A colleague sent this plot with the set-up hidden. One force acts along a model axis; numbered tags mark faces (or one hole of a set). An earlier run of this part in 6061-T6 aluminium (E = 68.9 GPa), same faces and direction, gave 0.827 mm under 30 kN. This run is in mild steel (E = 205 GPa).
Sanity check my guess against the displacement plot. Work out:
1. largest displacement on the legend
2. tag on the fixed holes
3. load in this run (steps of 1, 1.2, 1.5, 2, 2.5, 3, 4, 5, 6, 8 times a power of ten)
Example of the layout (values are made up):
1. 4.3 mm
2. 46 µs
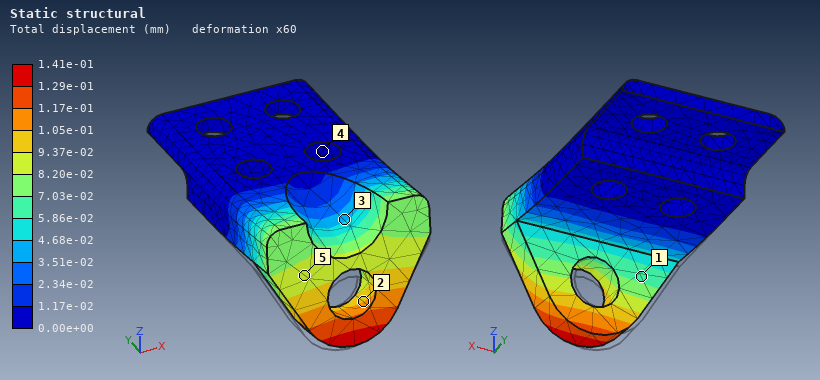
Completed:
1. 1.41e-01 mm
2. 4
3. 15 kN
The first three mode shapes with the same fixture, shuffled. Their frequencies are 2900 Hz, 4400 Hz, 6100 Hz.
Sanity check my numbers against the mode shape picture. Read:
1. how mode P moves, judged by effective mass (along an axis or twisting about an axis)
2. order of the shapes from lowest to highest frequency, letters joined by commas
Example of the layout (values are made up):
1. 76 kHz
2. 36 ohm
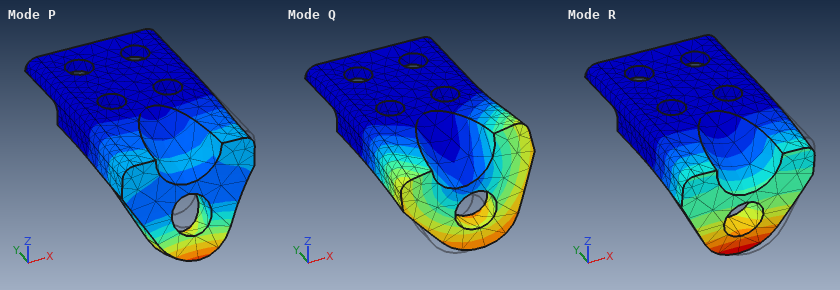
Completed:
1. along Z
2. R, Q, P
